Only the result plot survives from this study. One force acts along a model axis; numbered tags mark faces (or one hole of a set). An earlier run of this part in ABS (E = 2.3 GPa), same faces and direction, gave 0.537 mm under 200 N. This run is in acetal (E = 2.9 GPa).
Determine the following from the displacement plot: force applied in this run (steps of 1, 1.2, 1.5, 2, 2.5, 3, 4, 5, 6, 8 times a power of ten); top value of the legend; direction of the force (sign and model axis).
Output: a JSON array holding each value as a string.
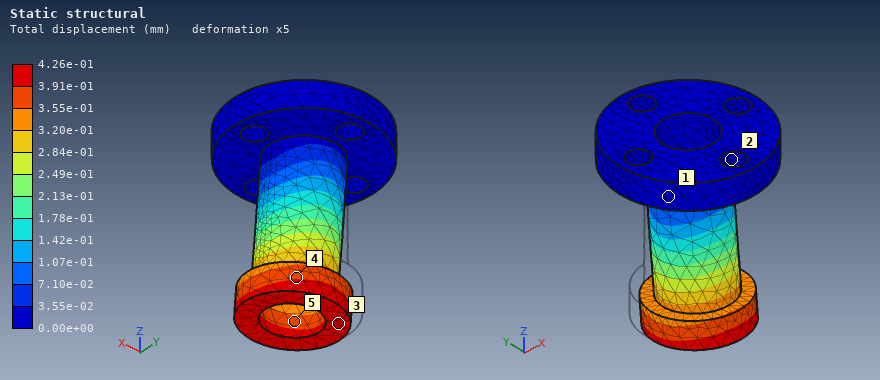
["200 N", "4.26e-01 mm", "-Y"]
